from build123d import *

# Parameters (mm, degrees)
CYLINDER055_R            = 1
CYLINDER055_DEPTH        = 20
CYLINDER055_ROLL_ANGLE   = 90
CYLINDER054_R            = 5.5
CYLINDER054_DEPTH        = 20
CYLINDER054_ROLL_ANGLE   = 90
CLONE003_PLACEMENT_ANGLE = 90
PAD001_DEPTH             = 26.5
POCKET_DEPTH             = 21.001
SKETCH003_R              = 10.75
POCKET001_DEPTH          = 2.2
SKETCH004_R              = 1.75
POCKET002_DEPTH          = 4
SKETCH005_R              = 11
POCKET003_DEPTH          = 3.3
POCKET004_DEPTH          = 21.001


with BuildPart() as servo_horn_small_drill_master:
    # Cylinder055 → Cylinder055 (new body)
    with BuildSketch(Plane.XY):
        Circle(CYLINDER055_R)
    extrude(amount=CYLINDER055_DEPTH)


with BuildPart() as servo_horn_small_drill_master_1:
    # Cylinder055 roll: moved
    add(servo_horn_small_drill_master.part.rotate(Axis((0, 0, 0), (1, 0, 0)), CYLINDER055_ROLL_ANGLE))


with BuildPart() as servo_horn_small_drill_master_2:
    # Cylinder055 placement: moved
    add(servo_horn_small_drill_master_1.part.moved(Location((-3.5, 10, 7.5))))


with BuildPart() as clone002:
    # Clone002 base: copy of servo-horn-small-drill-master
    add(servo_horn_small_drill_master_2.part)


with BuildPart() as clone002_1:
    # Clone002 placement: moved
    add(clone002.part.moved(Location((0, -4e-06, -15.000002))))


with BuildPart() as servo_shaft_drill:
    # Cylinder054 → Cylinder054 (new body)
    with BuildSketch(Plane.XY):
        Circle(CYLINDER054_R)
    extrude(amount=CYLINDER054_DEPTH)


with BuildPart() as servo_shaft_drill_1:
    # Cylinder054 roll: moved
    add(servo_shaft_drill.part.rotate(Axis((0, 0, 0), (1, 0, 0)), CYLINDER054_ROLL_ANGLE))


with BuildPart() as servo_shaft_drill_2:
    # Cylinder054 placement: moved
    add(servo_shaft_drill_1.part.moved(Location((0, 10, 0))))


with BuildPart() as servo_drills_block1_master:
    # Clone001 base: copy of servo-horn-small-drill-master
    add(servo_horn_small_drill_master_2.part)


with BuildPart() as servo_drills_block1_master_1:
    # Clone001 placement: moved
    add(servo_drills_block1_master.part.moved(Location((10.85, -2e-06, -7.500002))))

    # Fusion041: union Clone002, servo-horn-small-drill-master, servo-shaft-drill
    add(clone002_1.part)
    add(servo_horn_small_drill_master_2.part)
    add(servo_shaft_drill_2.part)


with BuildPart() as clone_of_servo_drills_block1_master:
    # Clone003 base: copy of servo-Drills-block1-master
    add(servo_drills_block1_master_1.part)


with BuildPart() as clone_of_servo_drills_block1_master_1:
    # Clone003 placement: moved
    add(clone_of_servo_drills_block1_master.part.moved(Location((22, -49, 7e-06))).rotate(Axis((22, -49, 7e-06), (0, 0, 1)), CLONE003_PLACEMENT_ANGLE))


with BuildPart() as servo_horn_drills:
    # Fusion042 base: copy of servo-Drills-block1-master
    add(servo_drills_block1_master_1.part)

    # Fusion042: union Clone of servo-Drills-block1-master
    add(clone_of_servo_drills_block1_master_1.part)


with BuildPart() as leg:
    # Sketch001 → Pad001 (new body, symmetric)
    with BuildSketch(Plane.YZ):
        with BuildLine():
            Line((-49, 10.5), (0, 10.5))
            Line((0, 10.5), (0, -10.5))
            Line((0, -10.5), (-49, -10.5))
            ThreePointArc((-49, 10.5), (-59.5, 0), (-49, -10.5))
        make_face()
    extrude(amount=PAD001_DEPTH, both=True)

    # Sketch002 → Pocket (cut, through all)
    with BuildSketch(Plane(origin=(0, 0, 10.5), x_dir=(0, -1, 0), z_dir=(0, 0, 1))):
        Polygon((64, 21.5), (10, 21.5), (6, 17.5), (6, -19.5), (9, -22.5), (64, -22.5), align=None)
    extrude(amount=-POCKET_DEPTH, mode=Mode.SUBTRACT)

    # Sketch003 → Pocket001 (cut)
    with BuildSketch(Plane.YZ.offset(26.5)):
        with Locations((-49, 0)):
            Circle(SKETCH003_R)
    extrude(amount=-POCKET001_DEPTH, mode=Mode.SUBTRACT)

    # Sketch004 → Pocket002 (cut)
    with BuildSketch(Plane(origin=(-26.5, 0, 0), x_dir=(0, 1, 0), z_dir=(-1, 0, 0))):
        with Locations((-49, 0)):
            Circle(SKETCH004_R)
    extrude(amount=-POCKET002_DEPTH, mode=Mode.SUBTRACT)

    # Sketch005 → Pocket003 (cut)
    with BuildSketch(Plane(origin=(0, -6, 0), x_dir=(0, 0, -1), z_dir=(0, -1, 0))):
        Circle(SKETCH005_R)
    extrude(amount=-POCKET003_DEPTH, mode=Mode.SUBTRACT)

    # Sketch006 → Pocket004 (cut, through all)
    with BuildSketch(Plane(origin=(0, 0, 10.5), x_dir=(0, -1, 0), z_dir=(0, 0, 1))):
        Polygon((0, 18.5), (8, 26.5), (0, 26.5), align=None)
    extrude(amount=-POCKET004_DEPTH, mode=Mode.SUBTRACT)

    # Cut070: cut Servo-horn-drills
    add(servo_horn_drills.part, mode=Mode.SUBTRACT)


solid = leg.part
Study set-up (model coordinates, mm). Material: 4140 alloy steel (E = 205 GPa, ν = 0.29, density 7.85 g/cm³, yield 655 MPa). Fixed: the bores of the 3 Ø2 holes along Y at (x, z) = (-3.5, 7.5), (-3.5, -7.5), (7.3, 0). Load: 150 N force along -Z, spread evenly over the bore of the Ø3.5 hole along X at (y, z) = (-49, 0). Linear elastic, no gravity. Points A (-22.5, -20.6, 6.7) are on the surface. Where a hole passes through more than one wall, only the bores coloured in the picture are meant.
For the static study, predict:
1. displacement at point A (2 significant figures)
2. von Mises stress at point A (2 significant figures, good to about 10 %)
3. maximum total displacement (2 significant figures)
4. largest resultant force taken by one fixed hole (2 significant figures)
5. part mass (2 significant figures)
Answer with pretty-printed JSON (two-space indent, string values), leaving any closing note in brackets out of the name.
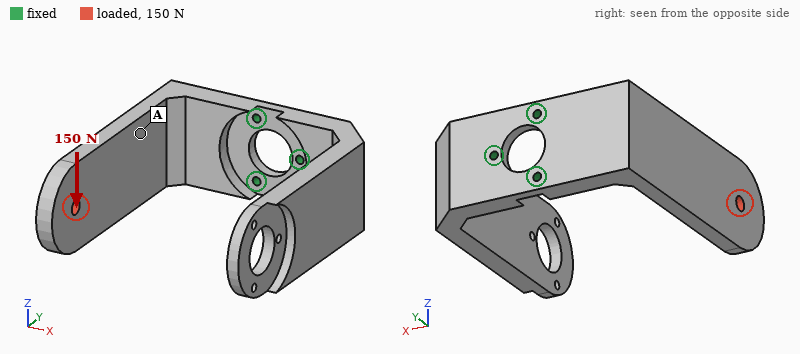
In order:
{
  "displacement at point A": "0.035 mm",
  "von Mises stress at point A": "12 MPa",
  "maximum total displacement": "0.11 mm",
  "largest resultant force taken by one fixed hole": "450 N",
  "part mass": "100 g"
}
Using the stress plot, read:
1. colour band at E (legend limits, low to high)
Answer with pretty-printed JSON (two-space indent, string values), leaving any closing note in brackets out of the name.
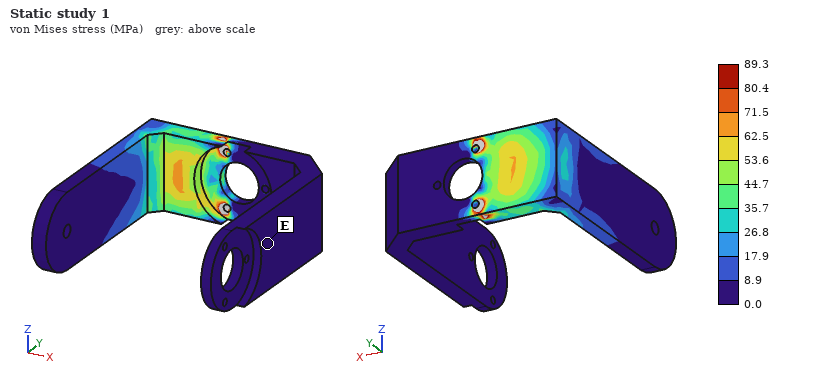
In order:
{
  "colour band at E": "0.0 to 8.9 MPa"
}
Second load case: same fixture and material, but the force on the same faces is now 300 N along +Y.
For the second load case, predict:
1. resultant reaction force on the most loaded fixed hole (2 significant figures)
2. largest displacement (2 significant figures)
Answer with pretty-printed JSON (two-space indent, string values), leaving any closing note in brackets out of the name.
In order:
{
  "resultant reaction force on the most loaded fixed hole": "170 N",
  "largest displacement": "0.31 mm"
}
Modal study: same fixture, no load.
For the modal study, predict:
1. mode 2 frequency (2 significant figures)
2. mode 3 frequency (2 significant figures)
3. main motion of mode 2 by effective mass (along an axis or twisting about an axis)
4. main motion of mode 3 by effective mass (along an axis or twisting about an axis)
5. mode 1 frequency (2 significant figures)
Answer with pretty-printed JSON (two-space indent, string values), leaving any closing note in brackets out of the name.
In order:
{
  "mode 2 frequency": "980 Hz",
  "mode 3 frequency": "1300 Hz",
  "main motion of mode 2 by effective mass": "along X",
  "main motion of mode 3 by effective mass": "along Z",
  "mode 1 frequency": "650 Hz"
}
